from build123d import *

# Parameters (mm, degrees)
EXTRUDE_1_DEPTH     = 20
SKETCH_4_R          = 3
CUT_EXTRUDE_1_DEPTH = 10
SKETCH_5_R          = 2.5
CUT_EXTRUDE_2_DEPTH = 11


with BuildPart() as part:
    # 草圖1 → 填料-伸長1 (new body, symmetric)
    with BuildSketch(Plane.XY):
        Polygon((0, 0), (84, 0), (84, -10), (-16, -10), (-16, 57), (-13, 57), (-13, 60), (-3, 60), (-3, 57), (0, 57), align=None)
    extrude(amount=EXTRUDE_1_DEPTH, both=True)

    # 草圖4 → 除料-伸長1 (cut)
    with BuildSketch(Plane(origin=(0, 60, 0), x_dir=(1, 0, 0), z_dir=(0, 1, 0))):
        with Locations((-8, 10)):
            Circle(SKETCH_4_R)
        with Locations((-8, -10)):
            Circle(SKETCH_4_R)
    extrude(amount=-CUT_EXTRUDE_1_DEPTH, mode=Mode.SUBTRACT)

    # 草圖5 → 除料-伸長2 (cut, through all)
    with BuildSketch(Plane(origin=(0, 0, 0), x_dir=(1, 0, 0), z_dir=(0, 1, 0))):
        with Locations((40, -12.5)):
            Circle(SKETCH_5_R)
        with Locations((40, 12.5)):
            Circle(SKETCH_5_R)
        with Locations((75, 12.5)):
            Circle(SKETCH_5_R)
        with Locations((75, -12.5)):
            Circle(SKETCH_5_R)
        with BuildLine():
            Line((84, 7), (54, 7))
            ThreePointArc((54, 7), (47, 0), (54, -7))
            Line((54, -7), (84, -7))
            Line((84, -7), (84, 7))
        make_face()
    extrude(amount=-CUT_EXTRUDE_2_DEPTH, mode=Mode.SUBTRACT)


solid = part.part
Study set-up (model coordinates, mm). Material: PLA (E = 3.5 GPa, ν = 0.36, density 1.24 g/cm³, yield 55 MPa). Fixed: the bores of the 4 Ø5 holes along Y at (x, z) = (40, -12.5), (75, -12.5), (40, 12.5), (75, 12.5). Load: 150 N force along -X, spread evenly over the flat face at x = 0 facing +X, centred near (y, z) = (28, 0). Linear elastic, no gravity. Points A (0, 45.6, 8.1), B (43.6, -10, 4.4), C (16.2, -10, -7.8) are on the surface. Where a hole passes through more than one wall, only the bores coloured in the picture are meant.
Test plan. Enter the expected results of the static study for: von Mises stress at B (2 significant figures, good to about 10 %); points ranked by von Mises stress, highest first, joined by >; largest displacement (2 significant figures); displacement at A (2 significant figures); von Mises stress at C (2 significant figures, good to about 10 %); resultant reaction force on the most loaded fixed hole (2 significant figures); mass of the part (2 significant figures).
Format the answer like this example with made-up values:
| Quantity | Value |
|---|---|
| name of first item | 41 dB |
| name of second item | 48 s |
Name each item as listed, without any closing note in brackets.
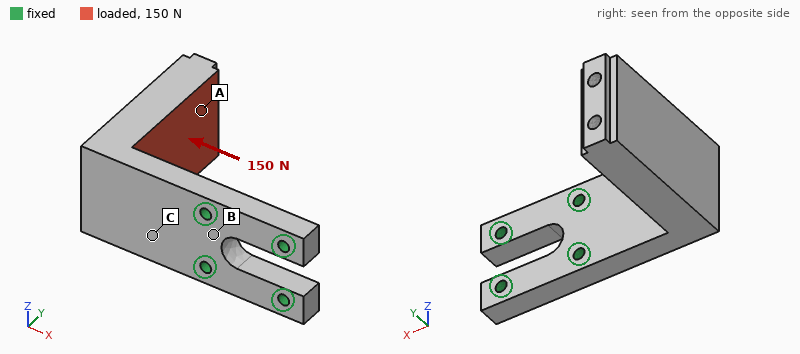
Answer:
| Quantity | Value |
|---|---|
| von Mises stress at B | 2.3 MPa |
| points ranked by von Mises stress, highest first, joined by > | C > B > A |
| largest displacement | 1.4 mm |
| displacement at A | 1.1 mm |
| von Mises stress at C | 6.7 MPa |
| resultant reaction force on the most loaded fixed hole | 73 N |
| mass of the part | 88 g |
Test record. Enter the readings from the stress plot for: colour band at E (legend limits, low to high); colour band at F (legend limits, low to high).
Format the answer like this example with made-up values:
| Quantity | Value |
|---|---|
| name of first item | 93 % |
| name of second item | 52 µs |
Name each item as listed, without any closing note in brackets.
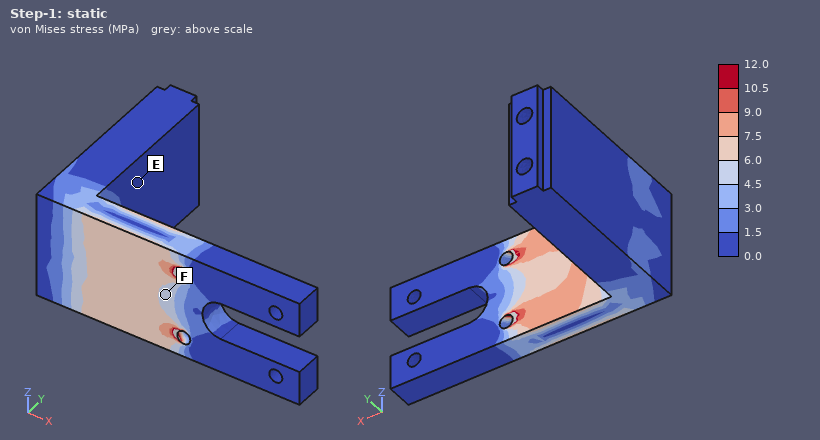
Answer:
| Quantity | Value |
|---|---|
| colour band at E | 0.0 to 1.5 MPa |
| colour band at F | 4.5 to 6.0 MPa |
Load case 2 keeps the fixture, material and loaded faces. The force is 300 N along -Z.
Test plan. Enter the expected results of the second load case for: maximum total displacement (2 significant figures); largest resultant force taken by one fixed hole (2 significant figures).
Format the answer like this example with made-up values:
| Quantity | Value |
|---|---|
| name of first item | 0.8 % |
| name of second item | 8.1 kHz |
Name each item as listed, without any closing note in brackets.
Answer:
| Quantity | Value |
|---|---|
| maximum total displacement | 1.5 mm |
| largest resultant force taken by one fixed hole | 540 N |
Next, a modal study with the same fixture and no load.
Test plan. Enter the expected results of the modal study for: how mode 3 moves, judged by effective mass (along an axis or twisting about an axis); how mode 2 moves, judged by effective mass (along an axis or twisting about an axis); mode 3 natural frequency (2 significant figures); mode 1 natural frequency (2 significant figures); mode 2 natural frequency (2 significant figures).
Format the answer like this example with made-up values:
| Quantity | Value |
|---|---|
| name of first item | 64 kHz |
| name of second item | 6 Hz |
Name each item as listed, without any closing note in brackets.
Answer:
| Quantity | Value |
|---|---|
| how mode 3 moves, judged by effective mass | along Y |
| how mode 2 moves, judged by effective mass | along Z |
| mode 3 natural frequency | 880 Hz |
| mode 1 natural frequency | 240 Hz |
| mode 2 natural frequency | 400 Hz |
